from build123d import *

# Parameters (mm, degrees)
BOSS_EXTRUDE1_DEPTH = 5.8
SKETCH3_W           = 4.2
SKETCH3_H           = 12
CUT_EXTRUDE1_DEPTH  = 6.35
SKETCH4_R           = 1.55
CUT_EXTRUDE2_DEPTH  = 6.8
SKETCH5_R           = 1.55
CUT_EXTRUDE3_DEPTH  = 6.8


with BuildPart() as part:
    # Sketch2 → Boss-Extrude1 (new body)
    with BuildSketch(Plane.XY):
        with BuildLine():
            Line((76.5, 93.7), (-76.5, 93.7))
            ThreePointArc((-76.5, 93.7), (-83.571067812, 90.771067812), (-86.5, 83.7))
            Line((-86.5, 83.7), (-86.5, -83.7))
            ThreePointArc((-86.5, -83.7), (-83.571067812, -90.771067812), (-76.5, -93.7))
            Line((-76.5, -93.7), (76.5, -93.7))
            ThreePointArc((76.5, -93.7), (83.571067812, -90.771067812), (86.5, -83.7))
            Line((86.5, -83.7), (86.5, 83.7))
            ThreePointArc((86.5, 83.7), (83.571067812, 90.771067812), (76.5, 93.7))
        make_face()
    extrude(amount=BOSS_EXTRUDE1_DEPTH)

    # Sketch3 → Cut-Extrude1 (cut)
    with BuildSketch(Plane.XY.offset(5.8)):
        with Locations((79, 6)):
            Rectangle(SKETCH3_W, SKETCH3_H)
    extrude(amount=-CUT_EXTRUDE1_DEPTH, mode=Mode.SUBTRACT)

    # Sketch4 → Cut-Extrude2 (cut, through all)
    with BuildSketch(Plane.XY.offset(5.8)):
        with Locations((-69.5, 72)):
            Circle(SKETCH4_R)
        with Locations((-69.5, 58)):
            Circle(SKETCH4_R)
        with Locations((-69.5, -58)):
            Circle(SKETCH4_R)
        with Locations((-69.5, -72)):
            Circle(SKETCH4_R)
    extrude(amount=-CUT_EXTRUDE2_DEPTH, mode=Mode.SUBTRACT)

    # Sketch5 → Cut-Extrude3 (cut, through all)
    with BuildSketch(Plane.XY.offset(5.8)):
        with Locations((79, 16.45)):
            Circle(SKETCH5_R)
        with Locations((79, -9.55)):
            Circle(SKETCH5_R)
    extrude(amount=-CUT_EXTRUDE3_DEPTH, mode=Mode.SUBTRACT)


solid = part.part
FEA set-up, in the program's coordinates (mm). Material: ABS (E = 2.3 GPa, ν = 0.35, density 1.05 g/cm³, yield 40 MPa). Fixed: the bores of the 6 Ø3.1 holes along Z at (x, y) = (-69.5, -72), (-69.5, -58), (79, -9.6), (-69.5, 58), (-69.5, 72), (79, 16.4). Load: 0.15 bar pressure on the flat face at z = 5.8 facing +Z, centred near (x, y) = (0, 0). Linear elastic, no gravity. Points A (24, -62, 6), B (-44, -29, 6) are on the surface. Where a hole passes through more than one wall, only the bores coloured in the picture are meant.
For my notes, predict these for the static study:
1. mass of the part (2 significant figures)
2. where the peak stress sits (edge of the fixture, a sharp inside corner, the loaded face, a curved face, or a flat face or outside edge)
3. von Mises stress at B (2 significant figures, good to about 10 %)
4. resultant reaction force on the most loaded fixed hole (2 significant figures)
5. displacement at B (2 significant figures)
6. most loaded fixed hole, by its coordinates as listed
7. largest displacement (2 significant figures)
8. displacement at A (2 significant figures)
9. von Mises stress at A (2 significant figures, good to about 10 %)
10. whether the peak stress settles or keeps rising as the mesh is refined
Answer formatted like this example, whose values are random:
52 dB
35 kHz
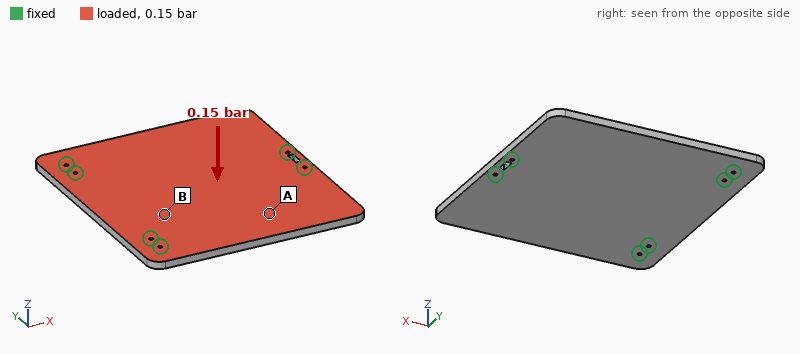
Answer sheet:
200 g
edge of the fixture
1.6 MPa
120 N
0.52 mm
(79, -9.6)
2.4 mm
1.6 mm
3.9 MPa
keeps rising
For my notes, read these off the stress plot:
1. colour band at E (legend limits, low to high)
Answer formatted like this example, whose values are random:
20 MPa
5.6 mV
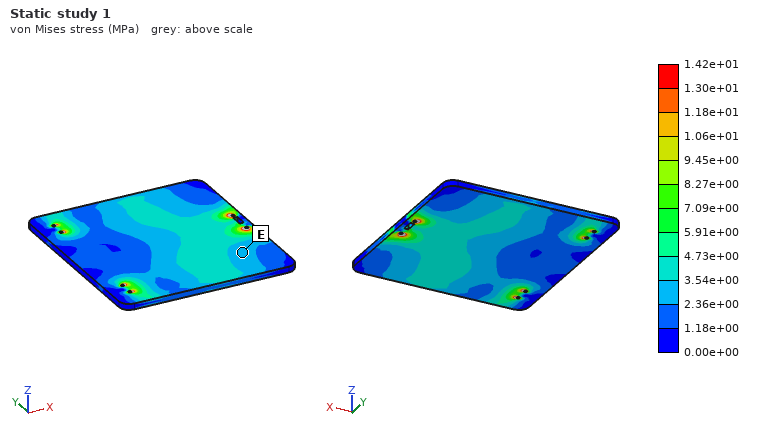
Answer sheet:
2.36e+00 to 3.54e+00 MPa
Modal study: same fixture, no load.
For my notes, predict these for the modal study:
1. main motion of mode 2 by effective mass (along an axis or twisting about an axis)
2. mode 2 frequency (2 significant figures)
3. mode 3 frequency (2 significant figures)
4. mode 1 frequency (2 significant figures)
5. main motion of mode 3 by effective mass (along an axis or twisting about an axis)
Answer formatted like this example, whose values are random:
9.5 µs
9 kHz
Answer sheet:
along Z
220 Hz
360 Hz
200 Hz
along Z
